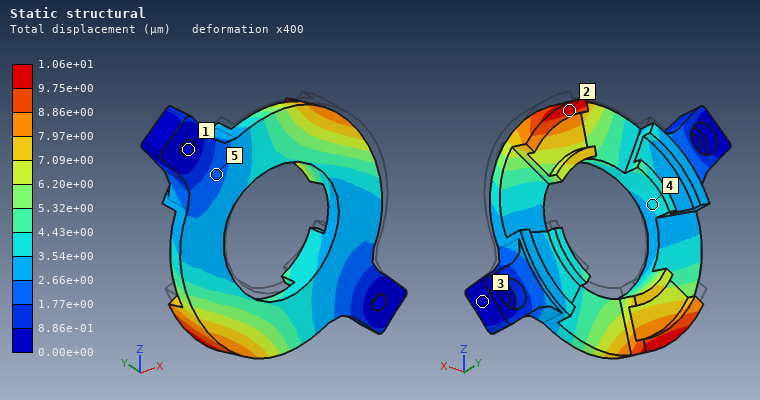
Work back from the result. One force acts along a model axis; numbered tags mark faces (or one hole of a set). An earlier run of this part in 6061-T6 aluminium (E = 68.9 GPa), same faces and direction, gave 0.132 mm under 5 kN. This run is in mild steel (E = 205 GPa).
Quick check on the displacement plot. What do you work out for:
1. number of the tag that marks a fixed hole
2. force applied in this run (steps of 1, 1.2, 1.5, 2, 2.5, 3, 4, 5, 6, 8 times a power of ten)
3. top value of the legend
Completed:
1
1.2 kN
1.06e+01 µm
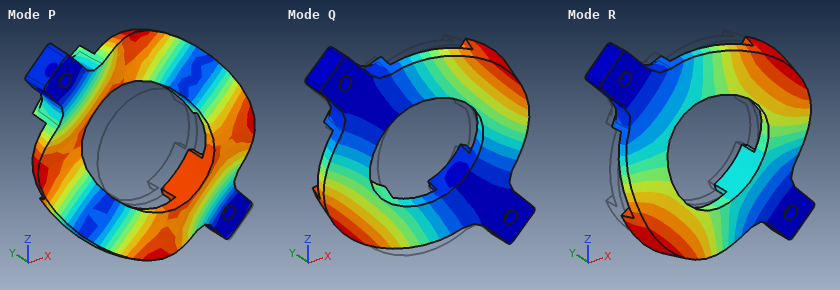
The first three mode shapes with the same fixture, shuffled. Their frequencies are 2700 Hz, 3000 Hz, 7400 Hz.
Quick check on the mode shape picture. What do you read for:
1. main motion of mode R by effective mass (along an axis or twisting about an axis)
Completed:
along Y
